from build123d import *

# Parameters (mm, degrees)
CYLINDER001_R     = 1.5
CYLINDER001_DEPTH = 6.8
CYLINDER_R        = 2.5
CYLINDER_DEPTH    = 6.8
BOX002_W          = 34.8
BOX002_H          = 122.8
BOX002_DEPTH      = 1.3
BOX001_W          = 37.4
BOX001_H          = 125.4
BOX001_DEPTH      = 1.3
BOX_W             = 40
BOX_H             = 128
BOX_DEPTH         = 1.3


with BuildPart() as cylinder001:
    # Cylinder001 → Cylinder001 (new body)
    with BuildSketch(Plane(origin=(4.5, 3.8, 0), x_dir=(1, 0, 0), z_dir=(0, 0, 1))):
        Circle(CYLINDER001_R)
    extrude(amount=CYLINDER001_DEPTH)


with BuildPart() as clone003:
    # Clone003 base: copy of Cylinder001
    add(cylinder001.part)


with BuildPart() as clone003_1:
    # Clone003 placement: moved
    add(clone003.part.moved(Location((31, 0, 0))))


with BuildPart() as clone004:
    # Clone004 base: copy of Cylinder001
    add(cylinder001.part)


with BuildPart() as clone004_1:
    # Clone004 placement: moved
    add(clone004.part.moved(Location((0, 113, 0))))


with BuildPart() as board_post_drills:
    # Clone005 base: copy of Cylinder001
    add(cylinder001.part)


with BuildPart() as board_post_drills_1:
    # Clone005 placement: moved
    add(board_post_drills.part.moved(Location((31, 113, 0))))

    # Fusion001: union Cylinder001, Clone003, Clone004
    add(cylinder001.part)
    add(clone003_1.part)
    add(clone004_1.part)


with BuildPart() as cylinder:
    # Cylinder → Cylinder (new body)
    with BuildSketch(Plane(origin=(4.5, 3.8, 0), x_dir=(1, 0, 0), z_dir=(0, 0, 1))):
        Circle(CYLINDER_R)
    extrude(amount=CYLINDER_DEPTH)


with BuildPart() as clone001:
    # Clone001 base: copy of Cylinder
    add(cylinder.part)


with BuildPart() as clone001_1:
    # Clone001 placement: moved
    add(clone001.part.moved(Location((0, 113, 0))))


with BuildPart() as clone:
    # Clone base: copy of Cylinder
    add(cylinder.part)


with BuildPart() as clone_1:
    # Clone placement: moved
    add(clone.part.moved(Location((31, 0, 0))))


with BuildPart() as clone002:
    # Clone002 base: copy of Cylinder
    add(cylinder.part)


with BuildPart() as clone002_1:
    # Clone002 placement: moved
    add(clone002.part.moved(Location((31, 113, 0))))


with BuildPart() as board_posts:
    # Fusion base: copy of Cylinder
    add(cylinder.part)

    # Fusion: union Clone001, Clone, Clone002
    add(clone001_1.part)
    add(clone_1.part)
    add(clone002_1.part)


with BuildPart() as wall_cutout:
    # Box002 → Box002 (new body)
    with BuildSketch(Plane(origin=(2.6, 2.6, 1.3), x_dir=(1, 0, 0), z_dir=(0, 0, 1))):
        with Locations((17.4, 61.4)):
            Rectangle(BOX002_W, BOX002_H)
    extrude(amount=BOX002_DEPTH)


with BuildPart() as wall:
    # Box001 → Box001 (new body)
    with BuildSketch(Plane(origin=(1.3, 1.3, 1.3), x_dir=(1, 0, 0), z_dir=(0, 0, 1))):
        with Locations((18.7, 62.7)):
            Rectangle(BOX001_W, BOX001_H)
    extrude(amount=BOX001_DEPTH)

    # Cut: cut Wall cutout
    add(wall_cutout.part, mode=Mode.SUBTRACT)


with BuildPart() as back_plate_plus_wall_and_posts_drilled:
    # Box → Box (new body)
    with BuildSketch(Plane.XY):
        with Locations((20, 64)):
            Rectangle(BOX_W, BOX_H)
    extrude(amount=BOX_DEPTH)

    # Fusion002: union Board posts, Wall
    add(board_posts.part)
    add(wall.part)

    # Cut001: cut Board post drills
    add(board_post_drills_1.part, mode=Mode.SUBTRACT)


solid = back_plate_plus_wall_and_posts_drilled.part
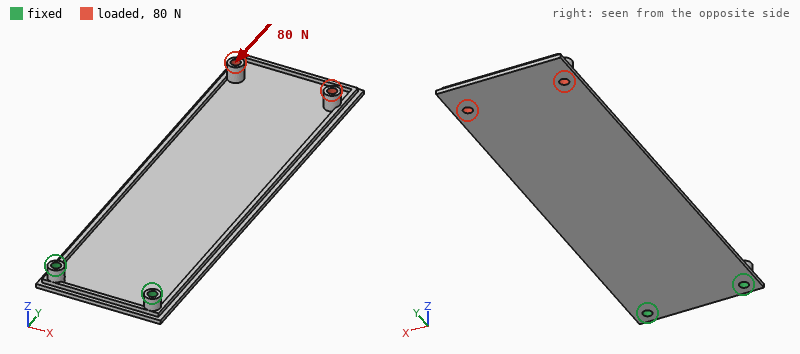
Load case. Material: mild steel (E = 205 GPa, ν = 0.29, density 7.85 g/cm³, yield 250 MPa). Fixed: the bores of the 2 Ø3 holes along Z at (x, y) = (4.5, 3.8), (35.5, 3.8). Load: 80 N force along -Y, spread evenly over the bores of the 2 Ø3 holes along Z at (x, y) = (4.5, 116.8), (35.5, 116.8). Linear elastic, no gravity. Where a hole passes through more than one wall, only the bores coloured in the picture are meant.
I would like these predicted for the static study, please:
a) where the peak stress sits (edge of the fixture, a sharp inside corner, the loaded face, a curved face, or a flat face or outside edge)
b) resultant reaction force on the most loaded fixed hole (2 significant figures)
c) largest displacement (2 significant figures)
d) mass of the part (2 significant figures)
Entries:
a flat face or outside edge
40 N
0.60 mm
58 g
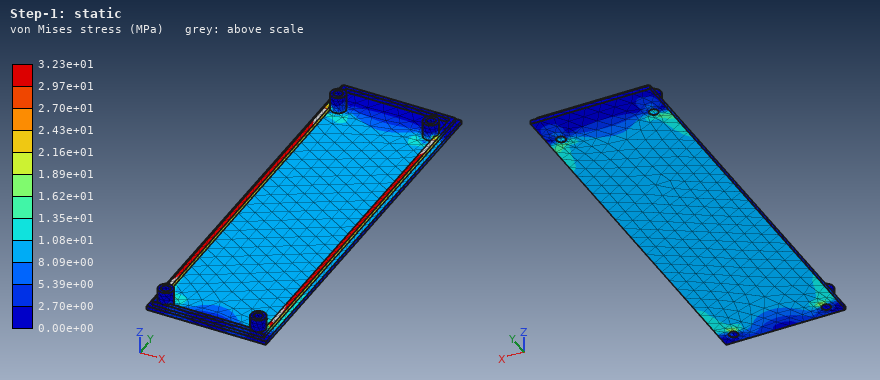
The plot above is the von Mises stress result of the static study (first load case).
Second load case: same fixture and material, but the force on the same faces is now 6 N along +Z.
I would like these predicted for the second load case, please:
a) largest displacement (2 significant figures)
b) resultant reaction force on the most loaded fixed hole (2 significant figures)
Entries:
1.2 mm
24 N
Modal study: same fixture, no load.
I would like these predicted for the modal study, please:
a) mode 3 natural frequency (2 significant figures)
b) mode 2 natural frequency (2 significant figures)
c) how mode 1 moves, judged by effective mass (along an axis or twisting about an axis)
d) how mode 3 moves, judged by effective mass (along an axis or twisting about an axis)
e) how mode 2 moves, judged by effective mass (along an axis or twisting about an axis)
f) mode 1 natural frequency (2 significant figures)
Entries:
560 Hz
450 Hz
along Z
along Z
twisting about Y
87 Hz
